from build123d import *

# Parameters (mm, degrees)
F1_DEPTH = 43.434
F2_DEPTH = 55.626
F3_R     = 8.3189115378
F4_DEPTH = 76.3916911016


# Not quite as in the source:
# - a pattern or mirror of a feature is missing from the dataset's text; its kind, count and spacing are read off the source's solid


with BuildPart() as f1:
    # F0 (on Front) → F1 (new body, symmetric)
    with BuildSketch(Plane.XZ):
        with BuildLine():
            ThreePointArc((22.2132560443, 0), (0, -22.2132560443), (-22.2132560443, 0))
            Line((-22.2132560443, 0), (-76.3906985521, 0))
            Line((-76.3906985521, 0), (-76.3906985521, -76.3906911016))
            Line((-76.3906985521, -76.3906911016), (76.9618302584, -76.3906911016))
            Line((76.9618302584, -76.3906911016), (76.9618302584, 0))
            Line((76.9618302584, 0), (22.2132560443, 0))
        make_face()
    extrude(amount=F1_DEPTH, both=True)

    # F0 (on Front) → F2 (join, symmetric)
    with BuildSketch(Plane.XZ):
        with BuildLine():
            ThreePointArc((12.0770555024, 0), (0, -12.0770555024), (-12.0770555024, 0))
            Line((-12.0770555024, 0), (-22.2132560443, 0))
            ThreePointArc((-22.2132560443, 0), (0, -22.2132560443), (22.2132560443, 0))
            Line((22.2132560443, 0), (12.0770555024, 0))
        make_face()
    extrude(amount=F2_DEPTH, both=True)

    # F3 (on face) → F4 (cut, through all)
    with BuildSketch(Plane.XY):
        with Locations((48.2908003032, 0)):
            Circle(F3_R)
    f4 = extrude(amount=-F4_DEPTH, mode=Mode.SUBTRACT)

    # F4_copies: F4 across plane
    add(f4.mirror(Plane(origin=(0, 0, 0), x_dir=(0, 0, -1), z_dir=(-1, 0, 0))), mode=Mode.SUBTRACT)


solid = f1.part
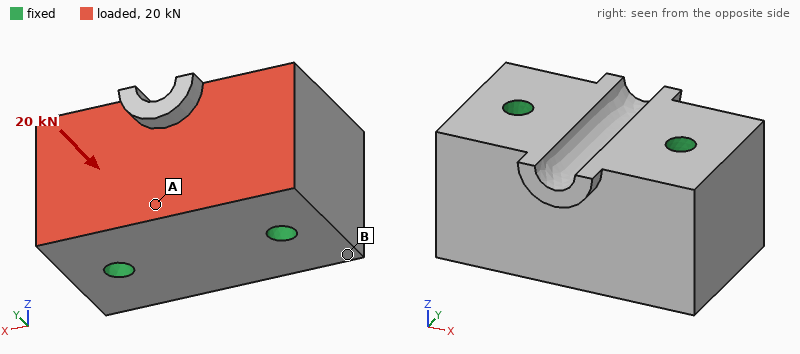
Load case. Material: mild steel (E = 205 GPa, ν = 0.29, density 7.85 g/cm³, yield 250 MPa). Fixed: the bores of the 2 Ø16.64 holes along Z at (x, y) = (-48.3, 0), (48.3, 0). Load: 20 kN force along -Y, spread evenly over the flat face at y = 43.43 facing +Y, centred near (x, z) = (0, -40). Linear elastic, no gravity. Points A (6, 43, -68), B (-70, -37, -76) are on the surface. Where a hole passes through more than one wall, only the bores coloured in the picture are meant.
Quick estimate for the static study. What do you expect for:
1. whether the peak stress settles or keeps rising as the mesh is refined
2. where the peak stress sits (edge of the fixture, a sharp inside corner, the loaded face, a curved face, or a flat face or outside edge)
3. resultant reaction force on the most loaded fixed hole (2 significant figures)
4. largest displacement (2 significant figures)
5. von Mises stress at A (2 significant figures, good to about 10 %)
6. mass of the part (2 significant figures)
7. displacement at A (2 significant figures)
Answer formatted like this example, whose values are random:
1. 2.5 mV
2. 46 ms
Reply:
1. keeps rising
2. edge of the fixture
3. 10 kN
4. 0.74 µm
5. 1.6 MPa
6. 7.7 kg
7. 0.69 µm
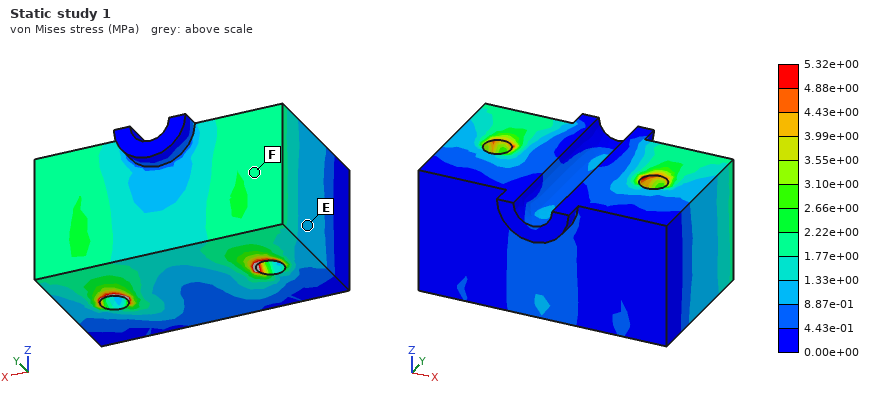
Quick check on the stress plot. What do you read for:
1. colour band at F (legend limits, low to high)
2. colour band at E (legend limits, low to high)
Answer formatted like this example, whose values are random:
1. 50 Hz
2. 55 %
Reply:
1. 1.77e+00 to 2.22e+00 MPa
2. 8.87e-01 to 1.33e+00 MPa
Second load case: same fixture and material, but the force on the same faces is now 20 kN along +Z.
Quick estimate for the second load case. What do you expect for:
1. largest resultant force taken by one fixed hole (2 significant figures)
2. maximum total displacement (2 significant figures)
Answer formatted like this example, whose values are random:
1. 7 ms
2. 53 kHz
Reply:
1. 10 kN
2. 2.8 µm
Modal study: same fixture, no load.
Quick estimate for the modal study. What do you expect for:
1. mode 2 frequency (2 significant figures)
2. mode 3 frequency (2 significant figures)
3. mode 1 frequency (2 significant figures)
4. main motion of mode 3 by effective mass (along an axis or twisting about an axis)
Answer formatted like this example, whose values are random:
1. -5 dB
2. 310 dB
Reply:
1. 12 kHz
2. 12 kHz
3. 11 kHz
4. along Y
